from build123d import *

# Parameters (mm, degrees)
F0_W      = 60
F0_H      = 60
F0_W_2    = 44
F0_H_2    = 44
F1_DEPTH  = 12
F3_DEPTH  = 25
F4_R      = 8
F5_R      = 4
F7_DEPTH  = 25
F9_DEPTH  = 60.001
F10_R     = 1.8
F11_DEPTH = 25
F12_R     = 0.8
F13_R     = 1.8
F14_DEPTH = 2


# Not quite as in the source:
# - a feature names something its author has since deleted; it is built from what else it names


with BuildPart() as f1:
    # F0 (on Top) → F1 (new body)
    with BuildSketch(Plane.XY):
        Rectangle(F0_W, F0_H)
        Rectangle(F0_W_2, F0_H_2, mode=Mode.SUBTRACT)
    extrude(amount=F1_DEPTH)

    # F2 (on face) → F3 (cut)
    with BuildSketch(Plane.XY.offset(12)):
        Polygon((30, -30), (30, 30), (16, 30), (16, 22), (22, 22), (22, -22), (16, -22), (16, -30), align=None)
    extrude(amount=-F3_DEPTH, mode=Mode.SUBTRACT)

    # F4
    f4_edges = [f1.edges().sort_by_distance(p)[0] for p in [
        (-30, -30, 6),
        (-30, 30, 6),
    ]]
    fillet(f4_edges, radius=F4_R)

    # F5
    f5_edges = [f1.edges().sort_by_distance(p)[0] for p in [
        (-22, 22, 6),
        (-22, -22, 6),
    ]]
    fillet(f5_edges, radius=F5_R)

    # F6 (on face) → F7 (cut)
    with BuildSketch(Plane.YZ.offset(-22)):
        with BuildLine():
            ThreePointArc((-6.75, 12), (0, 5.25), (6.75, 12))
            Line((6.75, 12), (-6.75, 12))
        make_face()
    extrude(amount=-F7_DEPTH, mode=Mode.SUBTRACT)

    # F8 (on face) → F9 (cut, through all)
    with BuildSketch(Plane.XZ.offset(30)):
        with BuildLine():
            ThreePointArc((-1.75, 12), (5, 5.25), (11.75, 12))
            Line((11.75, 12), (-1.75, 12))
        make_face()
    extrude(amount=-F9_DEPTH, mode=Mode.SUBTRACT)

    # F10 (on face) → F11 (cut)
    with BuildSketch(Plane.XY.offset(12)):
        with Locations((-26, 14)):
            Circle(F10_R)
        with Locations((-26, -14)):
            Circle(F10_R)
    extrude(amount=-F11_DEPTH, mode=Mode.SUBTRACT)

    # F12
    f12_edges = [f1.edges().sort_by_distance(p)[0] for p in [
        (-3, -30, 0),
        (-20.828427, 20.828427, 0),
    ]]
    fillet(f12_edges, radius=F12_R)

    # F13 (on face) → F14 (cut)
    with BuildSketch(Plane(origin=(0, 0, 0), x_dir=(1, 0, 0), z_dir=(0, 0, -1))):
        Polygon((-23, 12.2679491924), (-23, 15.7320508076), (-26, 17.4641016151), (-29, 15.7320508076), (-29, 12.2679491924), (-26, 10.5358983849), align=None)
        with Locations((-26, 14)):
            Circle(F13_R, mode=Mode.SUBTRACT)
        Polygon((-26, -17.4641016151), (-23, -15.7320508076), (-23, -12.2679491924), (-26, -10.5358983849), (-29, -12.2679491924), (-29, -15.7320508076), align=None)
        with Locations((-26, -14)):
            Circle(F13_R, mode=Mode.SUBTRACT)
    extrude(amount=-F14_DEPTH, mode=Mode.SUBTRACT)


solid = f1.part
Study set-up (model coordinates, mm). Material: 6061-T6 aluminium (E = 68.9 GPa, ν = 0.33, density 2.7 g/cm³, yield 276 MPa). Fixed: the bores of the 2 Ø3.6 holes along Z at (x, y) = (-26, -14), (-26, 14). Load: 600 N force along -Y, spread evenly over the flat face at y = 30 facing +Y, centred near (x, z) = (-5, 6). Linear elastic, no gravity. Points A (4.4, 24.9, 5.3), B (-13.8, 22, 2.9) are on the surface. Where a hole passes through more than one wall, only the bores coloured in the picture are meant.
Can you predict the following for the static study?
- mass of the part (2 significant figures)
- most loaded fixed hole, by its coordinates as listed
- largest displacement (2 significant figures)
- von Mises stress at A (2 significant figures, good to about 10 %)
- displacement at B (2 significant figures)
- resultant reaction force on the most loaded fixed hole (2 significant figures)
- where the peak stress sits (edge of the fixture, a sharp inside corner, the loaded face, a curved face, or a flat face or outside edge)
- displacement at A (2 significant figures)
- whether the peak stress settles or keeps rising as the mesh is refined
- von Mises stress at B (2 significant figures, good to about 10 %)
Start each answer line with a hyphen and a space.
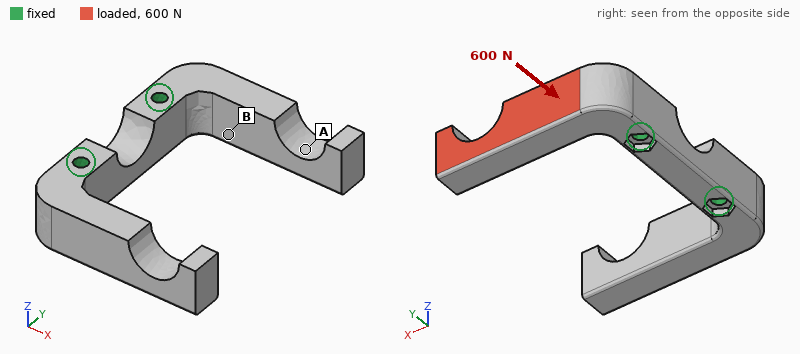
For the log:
- 29 g
- (-26, 14)
- 0.30 mm
- 25 MPa
- 0.060 mm
- 600 N
- edge of the fixture
- 0.19 mm
- keeps rising
- 48 MPa
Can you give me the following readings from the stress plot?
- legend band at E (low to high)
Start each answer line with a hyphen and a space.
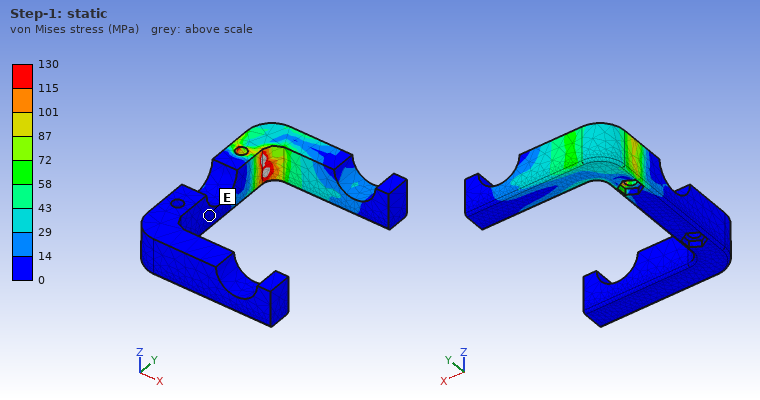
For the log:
- 0 to 14 MPa
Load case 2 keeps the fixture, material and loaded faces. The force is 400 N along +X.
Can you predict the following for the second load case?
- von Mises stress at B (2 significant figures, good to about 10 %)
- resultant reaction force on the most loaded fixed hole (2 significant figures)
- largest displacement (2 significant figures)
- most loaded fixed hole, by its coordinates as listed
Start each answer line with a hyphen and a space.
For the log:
- 5.8 MPa
- 440 N
- 94 µm
- (-26, 14)
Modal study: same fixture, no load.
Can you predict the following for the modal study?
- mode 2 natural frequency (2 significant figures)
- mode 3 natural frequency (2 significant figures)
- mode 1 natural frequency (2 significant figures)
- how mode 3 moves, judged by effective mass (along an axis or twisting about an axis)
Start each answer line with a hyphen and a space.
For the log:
- 3000 Hz
- 3500 Hz
- 3000 Hz
- along Z
